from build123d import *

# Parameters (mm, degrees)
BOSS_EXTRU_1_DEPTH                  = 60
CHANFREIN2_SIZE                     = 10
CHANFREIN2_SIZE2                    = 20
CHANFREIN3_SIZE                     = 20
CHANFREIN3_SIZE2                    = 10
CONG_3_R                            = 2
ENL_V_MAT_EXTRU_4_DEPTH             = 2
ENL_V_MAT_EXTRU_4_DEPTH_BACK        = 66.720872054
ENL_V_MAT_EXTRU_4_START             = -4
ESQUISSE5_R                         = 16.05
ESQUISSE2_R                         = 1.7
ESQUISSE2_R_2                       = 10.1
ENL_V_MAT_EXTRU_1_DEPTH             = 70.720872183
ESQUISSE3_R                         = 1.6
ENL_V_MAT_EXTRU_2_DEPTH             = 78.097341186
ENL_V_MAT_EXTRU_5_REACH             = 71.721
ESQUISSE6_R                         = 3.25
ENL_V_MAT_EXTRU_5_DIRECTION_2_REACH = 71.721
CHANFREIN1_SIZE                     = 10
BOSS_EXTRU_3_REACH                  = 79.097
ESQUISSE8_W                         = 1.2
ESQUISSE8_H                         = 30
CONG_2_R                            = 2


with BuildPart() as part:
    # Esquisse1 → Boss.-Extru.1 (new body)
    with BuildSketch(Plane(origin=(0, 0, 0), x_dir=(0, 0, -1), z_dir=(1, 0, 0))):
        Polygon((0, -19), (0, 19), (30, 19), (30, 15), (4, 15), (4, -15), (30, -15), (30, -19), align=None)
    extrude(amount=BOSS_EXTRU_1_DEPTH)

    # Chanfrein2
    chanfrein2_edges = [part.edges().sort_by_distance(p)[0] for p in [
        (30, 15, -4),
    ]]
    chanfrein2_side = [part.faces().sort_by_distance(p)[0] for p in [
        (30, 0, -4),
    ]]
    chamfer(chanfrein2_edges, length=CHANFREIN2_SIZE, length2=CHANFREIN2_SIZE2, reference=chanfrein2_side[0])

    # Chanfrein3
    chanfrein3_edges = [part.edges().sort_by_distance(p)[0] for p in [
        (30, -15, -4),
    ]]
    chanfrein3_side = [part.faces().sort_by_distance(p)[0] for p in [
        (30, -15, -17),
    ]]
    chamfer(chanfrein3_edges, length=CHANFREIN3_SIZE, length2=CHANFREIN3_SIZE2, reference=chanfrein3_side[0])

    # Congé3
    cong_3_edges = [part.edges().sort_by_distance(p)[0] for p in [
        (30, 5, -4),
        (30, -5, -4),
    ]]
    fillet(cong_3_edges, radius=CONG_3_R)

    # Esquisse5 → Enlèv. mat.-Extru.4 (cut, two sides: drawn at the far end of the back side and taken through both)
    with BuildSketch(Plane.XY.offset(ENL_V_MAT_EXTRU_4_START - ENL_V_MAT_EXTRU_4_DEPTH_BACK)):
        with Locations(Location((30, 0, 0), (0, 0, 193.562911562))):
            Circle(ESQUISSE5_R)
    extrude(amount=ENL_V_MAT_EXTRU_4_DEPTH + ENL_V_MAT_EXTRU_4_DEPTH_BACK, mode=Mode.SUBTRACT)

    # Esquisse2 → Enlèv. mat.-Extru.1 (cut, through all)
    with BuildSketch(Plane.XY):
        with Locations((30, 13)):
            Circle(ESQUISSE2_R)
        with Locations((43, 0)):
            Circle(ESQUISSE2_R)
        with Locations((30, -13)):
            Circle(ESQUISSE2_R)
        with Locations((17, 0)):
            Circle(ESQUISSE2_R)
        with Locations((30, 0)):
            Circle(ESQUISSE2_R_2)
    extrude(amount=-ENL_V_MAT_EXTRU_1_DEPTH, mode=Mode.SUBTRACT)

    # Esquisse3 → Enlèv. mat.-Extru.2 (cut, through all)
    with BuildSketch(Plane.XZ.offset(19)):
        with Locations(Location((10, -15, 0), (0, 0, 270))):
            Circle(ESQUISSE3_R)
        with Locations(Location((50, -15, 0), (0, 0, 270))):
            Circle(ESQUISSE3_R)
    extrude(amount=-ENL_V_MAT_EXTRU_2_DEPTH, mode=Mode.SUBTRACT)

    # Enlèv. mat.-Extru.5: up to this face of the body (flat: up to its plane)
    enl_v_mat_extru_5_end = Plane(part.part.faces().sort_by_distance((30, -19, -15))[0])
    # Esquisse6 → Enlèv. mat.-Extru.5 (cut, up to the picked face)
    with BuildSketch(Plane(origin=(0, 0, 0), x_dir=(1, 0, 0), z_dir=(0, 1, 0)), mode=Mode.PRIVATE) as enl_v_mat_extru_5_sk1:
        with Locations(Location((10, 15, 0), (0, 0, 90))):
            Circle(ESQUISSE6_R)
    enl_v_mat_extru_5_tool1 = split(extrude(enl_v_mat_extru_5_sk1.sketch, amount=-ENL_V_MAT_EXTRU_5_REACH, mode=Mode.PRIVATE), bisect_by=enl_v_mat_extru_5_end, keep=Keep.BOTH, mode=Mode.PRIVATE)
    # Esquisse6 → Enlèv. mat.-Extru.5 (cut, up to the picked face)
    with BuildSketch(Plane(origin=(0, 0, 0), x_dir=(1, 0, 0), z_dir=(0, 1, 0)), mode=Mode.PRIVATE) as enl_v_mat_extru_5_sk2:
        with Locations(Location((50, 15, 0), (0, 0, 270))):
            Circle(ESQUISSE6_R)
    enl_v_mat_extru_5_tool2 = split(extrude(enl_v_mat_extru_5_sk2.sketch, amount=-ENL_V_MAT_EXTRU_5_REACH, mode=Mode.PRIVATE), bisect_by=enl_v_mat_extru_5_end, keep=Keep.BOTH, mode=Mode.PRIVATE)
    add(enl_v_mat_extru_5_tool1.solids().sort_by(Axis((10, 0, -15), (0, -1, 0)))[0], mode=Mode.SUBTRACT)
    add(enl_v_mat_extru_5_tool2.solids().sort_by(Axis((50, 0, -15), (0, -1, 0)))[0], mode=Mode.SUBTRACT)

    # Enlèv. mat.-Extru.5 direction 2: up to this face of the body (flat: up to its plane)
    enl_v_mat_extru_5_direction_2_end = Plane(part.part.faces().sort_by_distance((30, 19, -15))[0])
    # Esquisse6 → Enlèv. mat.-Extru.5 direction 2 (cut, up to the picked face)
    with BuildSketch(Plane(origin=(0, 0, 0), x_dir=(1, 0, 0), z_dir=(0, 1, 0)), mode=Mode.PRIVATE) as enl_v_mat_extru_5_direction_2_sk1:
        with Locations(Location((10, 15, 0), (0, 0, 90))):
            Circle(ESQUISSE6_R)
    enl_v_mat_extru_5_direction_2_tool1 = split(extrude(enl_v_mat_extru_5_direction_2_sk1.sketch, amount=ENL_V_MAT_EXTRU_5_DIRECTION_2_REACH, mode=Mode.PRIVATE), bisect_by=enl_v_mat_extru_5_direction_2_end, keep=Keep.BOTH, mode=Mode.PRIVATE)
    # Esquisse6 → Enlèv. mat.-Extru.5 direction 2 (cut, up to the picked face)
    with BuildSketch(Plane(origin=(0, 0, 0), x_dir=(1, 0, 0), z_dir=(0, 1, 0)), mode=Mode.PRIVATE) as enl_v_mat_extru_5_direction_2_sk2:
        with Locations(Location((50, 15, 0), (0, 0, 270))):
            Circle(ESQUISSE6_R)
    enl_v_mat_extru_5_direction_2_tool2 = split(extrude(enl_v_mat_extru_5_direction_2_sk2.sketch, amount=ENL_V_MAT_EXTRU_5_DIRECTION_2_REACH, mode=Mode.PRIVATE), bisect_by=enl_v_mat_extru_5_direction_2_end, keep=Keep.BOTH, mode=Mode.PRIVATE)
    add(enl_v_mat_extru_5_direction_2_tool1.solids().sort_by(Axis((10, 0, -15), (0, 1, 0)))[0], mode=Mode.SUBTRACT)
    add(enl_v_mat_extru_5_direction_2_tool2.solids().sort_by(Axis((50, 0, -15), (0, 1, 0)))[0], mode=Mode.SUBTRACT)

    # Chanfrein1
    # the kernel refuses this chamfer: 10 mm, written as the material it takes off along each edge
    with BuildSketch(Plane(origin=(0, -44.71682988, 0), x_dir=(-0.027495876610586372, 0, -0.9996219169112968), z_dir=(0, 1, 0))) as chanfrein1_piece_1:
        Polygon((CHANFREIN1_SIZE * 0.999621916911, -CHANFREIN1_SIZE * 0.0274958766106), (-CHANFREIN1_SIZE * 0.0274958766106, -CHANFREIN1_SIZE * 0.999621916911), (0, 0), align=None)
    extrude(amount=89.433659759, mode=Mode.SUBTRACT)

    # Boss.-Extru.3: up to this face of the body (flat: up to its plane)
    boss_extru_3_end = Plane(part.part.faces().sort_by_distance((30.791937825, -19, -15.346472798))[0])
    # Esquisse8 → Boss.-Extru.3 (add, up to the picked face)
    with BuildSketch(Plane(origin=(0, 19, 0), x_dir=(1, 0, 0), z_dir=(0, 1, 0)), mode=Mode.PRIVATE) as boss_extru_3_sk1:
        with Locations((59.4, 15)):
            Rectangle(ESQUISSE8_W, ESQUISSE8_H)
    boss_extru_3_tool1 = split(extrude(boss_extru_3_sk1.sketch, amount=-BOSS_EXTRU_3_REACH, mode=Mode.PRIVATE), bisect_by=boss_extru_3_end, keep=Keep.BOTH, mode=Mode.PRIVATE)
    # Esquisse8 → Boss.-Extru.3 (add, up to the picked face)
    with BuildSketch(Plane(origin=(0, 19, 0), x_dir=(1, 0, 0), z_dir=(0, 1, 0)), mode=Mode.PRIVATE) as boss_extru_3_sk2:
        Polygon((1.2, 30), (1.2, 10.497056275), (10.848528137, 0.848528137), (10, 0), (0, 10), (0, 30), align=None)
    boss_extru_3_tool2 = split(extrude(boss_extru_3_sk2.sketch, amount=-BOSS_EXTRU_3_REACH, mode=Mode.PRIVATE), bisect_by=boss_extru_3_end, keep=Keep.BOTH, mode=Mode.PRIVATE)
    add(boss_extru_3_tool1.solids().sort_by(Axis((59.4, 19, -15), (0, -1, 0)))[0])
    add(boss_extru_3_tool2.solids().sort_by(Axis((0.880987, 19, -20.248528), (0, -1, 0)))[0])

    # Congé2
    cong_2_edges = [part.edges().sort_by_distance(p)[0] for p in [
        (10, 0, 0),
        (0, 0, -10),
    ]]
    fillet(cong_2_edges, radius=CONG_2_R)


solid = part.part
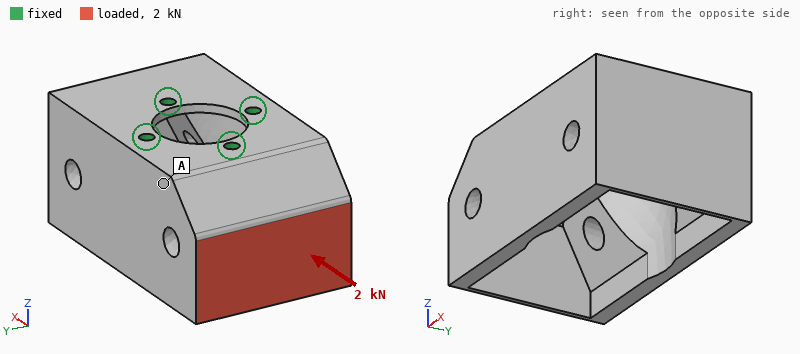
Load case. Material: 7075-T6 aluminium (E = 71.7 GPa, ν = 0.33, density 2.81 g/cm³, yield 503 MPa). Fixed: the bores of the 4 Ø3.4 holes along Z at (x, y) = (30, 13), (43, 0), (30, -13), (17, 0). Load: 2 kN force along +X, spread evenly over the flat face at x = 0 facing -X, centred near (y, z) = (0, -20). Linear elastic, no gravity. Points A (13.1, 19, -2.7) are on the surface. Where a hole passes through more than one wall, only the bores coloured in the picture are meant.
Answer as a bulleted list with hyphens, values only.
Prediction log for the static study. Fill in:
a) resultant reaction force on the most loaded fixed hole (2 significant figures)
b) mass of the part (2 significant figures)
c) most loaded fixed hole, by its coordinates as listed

- 1.3 kN
- 71 g
- (17, 0)
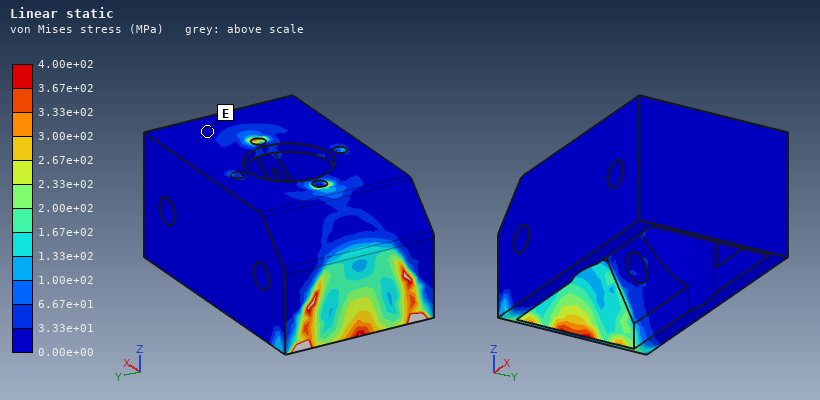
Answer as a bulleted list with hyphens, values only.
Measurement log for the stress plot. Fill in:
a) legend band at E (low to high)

- 0.00e+00 to 3.33e+01 MPa
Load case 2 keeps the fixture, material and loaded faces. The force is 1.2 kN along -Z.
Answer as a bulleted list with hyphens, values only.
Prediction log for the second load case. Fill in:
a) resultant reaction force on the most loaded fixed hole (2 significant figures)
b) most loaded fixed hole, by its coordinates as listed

- 1.5 kN
- (17, 0)
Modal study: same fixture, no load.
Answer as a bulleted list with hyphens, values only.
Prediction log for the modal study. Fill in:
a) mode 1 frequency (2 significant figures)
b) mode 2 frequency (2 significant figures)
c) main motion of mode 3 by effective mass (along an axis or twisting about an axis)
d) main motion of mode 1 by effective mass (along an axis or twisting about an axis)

- 3400 Hz
- 3800 Hz
- along Y
- along X
